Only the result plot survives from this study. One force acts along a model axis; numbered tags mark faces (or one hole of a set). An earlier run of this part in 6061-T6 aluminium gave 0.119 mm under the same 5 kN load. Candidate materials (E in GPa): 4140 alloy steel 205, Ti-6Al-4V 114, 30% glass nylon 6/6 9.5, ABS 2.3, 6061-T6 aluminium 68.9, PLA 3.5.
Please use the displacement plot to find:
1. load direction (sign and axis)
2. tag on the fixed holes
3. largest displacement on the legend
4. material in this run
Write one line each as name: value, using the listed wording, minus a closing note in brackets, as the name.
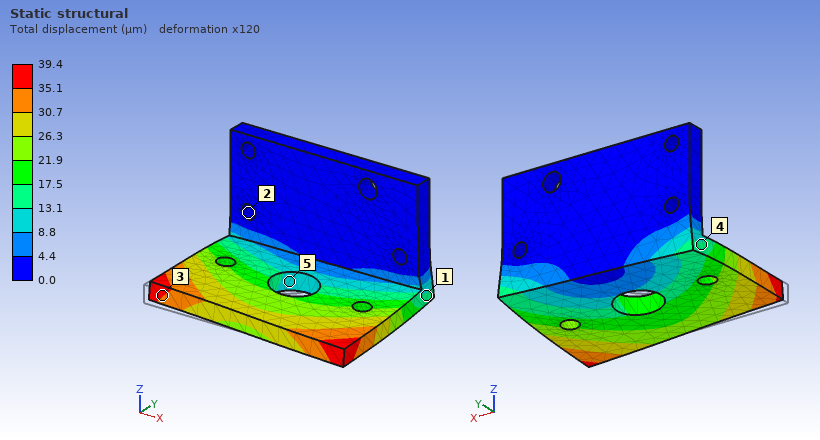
load direction: +X
tag on the fixed holes: 2
largest displacement on the legend: 39.4 µm
material in this run: 4140 alloy steel
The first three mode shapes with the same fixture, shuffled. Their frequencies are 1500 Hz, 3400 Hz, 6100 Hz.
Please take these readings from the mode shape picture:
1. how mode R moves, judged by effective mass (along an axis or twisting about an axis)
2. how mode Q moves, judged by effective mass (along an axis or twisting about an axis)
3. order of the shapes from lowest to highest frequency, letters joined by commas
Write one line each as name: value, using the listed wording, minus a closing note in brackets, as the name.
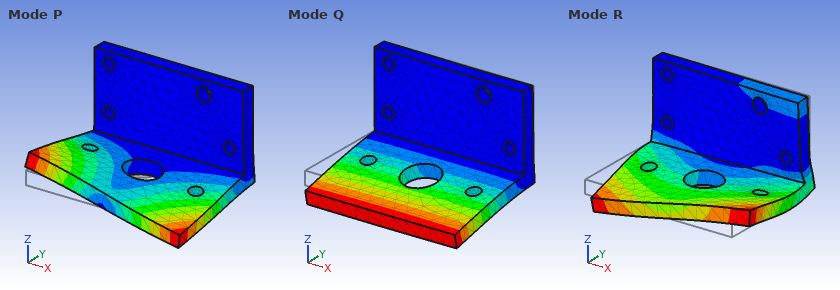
how mode R moves, judged by effective mass: along X
how mode Q moves, judged by effective mass: along Z
order of the shapes from lowest to highest frequency, letters joined by commas: Q, P, R
